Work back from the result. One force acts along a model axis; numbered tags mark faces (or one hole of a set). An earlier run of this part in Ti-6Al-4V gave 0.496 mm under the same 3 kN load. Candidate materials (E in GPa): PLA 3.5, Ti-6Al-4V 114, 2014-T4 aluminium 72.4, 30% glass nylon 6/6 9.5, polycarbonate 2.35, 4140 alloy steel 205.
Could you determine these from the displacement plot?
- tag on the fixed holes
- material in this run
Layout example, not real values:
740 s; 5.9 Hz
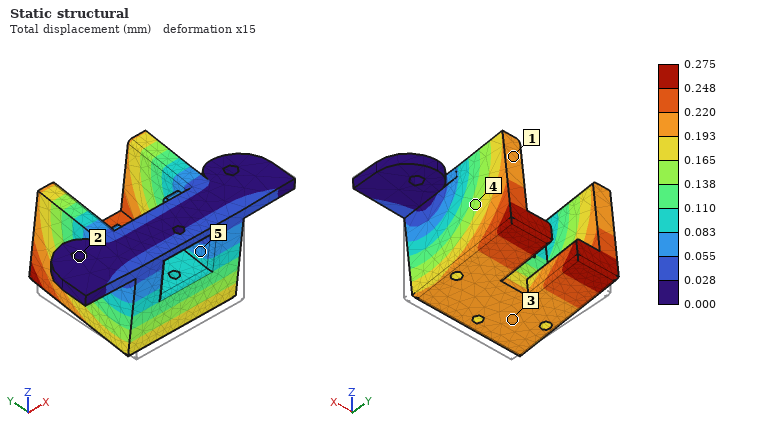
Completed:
2; 4140 alloy steel
